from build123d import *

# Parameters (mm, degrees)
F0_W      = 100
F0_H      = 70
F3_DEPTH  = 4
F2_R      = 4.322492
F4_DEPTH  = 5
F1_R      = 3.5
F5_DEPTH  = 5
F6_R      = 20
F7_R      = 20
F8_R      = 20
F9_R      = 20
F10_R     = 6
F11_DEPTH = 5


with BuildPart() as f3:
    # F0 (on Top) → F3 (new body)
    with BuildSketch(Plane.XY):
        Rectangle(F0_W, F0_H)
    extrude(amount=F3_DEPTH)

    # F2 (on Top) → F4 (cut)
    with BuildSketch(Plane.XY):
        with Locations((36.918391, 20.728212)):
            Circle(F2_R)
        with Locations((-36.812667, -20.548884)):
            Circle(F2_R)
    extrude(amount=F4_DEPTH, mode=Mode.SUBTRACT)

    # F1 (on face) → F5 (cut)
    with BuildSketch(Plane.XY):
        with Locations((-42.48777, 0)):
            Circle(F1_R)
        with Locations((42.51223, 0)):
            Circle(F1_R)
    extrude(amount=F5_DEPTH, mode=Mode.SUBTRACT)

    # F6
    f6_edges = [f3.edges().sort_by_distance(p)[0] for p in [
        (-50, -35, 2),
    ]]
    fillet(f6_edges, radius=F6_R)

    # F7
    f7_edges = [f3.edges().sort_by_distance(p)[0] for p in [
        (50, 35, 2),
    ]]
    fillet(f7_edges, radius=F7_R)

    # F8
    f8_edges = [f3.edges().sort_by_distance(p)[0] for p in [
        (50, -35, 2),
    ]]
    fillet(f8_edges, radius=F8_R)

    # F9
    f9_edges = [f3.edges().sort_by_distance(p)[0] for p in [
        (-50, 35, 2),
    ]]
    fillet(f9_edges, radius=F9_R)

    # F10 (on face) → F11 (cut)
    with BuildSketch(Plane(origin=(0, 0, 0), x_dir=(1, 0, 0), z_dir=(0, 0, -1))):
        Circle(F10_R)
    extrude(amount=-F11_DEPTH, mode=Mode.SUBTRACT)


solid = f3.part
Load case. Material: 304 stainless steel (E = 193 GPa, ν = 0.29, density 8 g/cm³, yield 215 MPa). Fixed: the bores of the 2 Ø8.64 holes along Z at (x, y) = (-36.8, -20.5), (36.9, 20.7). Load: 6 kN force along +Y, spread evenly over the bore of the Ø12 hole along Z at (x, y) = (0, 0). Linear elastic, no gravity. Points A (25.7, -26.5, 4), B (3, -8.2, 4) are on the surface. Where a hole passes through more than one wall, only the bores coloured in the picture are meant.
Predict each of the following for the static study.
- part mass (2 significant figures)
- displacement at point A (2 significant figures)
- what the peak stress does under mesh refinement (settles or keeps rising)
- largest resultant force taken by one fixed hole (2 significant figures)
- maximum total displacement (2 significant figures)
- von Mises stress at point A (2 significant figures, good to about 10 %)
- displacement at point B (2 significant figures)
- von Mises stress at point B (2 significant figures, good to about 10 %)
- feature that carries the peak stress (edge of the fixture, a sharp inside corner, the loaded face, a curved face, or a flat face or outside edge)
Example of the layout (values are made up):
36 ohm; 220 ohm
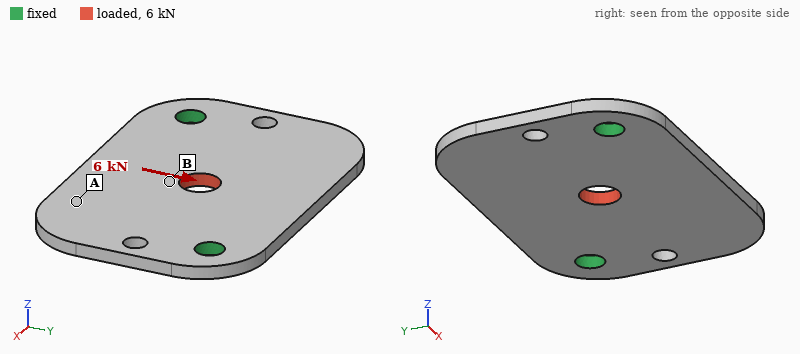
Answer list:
200 g; 6.2 µm; keeps rising; 3.0 kN; 11 µm; 13 MPa; 9.9 µm; 37 MPa; edge of the fixture
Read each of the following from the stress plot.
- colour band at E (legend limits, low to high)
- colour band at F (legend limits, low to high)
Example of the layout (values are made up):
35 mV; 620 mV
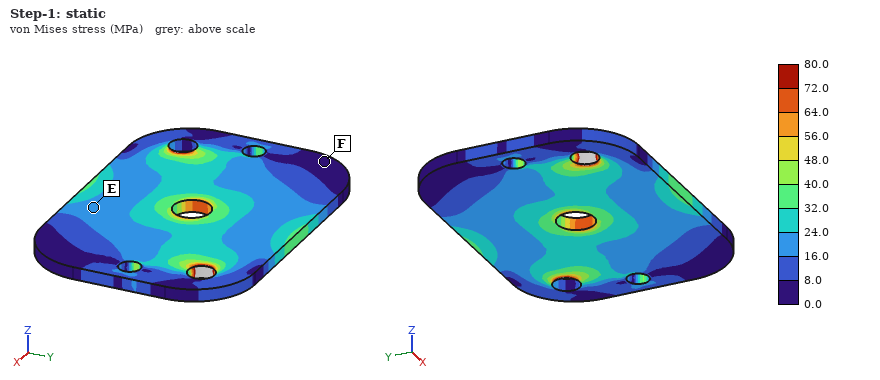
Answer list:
16.0 to 24.0 MPa; 0.0 to 8.0 MPa
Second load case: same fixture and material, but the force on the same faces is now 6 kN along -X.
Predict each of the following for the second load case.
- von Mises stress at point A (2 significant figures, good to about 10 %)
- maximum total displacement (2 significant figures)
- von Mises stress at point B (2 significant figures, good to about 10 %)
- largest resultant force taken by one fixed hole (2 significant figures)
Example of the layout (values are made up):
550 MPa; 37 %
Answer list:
8.4 MPa; 7.4 µm; 28 MPa; 3.0 kN
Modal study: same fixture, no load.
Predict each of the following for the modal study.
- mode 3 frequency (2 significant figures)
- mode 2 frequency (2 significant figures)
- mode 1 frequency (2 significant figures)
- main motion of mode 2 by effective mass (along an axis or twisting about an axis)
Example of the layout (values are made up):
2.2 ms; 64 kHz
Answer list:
3400 Hz; 1700 Hz; 1400 Hz; along Z
